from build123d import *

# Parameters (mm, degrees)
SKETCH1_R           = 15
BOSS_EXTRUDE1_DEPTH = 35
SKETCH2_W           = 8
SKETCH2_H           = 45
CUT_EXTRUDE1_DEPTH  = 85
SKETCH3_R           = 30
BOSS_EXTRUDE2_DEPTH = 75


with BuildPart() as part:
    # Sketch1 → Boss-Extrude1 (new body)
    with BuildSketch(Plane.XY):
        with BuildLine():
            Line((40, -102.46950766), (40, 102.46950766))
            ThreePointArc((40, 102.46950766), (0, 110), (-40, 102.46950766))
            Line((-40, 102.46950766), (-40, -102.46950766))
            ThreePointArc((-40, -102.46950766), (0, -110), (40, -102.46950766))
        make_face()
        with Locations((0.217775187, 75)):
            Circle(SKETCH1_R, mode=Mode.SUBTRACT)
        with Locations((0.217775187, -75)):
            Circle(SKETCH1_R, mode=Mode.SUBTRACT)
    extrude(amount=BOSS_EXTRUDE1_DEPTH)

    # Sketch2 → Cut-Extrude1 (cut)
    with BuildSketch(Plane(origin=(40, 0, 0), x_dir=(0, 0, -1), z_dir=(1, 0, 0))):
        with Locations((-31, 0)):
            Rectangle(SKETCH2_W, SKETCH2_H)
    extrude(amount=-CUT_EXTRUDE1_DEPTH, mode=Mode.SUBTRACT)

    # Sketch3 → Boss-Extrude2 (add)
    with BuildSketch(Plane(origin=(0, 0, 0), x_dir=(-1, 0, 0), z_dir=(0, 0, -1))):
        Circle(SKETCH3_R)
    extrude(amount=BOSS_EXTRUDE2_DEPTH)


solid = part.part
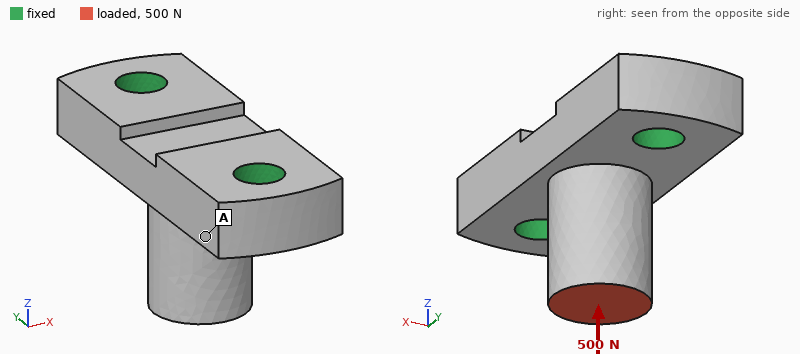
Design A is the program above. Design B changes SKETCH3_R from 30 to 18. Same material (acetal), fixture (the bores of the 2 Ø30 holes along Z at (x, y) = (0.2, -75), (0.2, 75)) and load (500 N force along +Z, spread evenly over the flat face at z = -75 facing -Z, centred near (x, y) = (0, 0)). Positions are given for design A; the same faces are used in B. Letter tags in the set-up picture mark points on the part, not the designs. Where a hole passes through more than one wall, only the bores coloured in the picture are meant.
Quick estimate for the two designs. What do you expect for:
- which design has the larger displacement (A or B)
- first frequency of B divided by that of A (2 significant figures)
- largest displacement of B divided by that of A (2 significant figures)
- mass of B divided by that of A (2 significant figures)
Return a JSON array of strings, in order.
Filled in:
["B", "1.1", "1.8", "0.82"]
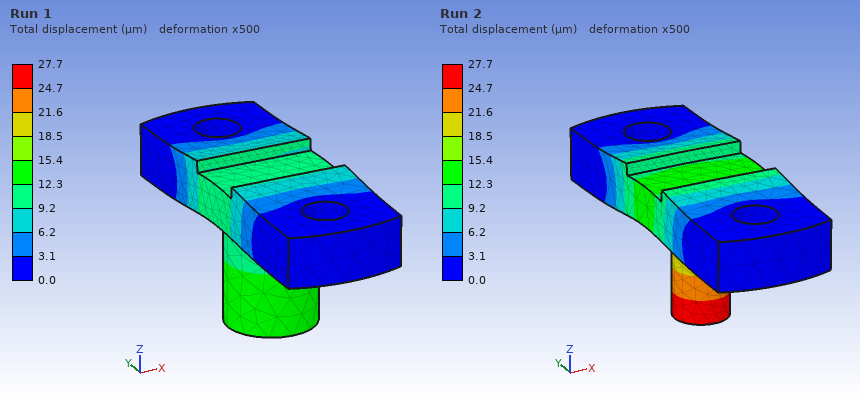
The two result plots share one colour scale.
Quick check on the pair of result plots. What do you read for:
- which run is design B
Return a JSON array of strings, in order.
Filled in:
["Run 2"]
